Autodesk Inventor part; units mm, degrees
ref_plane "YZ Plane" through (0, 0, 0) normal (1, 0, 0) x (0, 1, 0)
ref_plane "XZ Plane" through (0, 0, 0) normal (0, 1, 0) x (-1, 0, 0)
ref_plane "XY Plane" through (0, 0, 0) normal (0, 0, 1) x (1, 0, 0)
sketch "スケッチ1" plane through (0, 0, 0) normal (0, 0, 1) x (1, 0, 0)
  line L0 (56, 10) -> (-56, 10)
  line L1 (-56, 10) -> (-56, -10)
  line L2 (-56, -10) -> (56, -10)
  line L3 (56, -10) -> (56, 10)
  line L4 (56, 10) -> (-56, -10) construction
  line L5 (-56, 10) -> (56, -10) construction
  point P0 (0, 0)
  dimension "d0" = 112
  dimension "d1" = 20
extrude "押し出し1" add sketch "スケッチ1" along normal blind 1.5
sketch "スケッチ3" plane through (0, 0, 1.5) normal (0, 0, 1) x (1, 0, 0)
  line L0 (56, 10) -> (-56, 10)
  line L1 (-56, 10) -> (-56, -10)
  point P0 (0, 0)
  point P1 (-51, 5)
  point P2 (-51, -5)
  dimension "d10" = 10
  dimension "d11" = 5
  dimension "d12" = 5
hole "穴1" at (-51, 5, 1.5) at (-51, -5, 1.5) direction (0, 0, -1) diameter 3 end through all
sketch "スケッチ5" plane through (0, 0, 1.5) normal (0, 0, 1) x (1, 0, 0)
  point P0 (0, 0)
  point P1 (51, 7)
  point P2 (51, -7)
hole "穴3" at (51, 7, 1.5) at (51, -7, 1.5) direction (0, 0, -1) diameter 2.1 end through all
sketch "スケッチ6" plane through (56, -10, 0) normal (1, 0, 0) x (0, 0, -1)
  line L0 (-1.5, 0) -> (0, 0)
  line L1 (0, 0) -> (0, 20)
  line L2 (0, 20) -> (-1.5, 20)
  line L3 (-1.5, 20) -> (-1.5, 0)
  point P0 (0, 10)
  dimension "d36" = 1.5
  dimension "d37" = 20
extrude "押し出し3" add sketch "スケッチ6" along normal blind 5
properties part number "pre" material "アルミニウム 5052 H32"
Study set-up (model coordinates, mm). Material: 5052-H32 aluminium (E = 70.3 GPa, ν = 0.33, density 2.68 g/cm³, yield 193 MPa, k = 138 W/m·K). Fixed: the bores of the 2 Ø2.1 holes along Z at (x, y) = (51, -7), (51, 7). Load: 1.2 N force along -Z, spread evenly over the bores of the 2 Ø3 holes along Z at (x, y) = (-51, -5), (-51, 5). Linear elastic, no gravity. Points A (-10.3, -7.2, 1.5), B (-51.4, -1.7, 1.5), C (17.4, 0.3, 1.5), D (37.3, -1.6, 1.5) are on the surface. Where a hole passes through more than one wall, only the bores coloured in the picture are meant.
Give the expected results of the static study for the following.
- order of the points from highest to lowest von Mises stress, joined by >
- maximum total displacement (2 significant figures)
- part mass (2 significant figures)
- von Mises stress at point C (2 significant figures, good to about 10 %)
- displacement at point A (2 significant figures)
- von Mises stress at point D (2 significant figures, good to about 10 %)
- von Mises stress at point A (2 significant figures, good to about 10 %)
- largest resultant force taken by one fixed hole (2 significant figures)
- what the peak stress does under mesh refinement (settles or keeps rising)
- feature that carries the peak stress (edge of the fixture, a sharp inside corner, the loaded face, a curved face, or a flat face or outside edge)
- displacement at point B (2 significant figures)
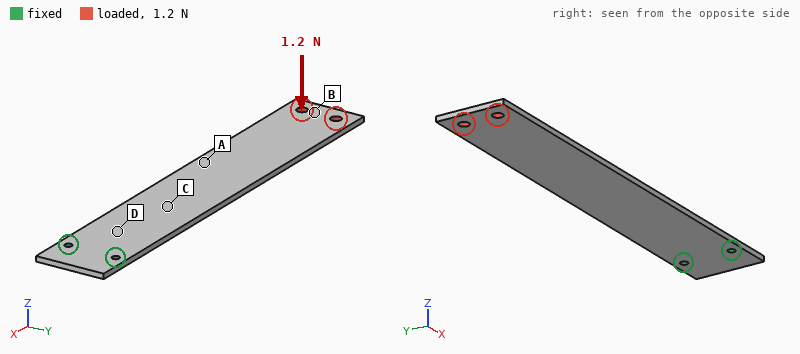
D > C > A > B
1.1 mm
9.3 g
11 MPa
0.46 mm
14 MPa
6.5 MPa
0.60 N
keeps rising
edge of the fixture
1.1 mm
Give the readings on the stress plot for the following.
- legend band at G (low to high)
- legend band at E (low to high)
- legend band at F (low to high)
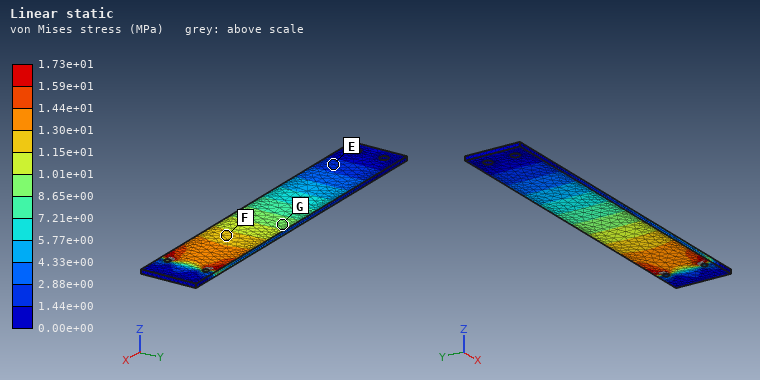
8.65e+00 to 1.01e+01 MPa
1.44e+00 to 2.88e+00 MPa
1.15e+01 to 1.30e+01 MPa
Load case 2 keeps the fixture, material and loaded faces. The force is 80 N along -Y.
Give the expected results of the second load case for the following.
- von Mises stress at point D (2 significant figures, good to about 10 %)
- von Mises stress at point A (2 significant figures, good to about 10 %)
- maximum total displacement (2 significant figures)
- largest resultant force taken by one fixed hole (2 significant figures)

13 MPa
24 MPa
0.45 mm
560 N
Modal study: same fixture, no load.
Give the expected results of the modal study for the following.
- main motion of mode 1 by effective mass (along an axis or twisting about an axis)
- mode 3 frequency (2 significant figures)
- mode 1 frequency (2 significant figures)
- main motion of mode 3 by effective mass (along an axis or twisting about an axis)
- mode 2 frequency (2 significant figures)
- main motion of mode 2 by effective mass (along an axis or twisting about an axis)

along Z
1100 Hz
110 Hz
twisting about X
690 Hz
along Z
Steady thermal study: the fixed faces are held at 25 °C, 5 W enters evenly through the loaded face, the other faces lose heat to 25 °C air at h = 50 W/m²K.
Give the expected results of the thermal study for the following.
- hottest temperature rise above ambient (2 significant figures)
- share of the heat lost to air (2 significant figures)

49 K
83 %
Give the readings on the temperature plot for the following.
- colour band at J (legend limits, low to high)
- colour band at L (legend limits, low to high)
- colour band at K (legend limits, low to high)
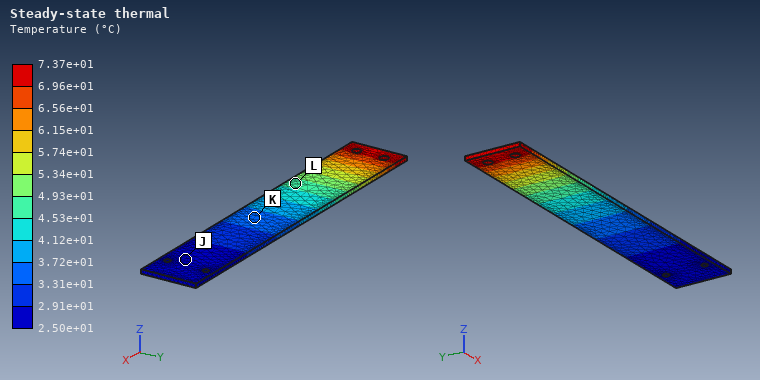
2.50e+01 to 2.91e+01 °C
4.53e+01 to 4.93e+01 °C
3.31e+01 to 3.72e+01 °C
